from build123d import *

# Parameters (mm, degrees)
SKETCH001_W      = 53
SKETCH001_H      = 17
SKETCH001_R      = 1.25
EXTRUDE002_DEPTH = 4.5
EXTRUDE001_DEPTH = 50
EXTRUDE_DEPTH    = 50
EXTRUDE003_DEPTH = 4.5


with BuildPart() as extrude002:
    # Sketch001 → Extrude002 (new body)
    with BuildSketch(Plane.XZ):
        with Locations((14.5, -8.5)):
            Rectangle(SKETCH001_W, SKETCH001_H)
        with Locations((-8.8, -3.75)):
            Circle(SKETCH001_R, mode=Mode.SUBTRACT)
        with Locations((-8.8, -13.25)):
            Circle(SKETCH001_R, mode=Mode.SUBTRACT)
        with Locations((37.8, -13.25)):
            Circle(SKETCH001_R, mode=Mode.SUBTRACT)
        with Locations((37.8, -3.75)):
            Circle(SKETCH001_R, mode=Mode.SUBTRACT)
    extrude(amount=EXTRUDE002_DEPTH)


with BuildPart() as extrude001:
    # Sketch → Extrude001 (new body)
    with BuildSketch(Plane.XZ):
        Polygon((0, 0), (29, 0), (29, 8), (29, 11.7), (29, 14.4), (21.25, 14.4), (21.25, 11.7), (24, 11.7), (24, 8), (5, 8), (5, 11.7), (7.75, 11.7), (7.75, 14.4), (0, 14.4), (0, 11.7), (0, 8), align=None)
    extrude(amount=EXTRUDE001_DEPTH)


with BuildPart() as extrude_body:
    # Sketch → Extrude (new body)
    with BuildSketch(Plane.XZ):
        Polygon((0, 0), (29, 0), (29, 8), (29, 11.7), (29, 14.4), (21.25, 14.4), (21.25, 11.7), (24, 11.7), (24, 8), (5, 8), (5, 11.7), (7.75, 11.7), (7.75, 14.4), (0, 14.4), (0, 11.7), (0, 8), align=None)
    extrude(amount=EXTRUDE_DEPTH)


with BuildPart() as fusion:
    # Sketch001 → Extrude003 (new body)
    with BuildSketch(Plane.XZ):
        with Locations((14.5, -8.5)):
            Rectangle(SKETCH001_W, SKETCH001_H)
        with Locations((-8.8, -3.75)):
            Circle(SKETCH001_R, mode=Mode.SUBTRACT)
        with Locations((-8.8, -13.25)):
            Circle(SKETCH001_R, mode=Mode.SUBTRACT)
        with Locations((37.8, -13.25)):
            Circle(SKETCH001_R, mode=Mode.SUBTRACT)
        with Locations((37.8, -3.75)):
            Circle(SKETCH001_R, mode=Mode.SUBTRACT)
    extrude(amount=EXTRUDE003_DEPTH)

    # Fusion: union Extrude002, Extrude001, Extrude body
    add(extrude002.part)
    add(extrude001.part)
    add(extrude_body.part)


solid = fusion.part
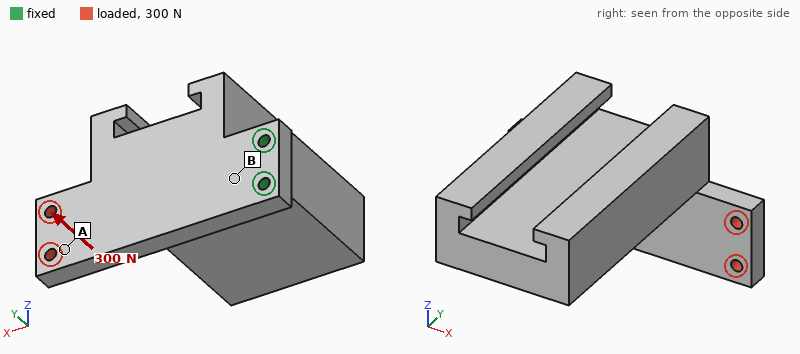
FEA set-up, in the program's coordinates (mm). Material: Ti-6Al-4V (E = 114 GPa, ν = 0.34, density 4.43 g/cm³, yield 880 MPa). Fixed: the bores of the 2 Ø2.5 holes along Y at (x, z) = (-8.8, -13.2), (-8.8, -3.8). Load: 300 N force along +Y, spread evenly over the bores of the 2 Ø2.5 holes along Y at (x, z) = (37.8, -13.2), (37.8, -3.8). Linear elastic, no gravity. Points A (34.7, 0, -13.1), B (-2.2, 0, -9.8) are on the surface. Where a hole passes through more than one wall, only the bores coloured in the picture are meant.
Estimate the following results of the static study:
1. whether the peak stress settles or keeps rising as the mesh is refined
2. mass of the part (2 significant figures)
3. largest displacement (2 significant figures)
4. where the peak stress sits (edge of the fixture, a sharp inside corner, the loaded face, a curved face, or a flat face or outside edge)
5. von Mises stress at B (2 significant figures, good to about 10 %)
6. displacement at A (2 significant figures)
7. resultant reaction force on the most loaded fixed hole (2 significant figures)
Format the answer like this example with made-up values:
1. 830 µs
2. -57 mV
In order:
1. keeps rising
2. 86 g
3. 0.68 mm
4. edge of the fixture
5. 180 MPa
6. 0.47 mm
7. 160 N
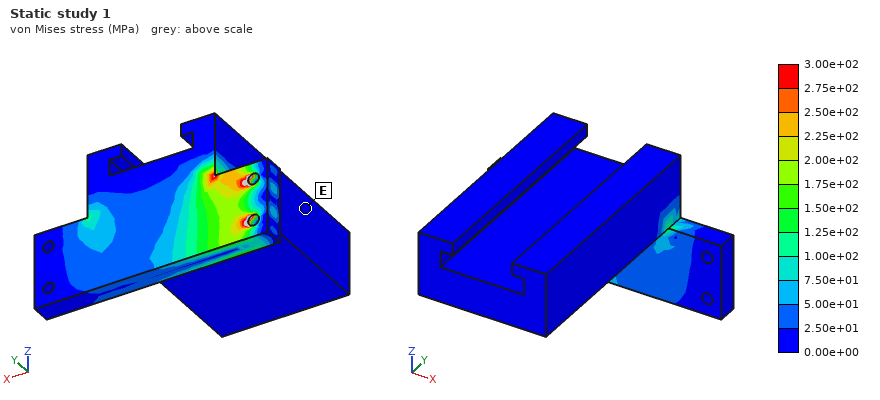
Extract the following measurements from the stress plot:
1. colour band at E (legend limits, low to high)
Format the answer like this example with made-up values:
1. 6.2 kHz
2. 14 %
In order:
1. 0.00e+00 to 2.50e+01 MPa
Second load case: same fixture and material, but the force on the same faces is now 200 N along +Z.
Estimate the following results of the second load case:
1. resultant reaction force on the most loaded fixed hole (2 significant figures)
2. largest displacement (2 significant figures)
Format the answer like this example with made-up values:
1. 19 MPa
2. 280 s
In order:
1. 850 N
2. 34 µm
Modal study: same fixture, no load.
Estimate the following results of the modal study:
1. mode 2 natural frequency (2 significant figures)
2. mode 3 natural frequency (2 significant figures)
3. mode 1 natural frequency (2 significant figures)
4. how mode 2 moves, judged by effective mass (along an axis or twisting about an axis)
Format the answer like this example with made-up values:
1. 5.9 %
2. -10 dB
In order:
1. 730 Hz
2. 3100 Hz
3. 520 Hz
4. along Z
